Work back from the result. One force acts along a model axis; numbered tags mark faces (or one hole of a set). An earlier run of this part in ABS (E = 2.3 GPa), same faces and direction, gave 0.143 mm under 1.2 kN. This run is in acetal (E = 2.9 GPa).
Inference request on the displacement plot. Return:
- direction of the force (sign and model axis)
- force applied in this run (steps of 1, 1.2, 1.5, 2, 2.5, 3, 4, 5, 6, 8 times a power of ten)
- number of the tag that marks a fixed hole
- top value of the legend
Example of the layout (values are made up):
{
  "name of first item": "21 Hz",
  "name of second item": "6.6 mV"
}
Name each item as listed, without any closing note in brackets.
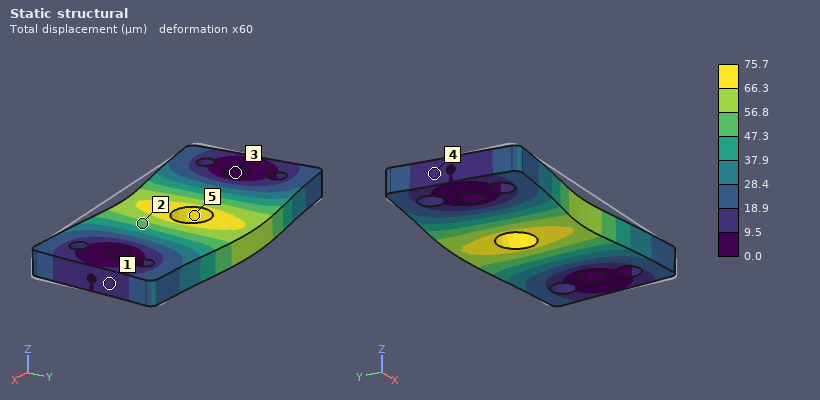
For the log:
{
  "direction of the force": "+Y",
  "force applied in this run": "800 N",
  "number of the tag that marks a fixed hole": "3",
  "top value of the legend": "75.7 µm"
}
